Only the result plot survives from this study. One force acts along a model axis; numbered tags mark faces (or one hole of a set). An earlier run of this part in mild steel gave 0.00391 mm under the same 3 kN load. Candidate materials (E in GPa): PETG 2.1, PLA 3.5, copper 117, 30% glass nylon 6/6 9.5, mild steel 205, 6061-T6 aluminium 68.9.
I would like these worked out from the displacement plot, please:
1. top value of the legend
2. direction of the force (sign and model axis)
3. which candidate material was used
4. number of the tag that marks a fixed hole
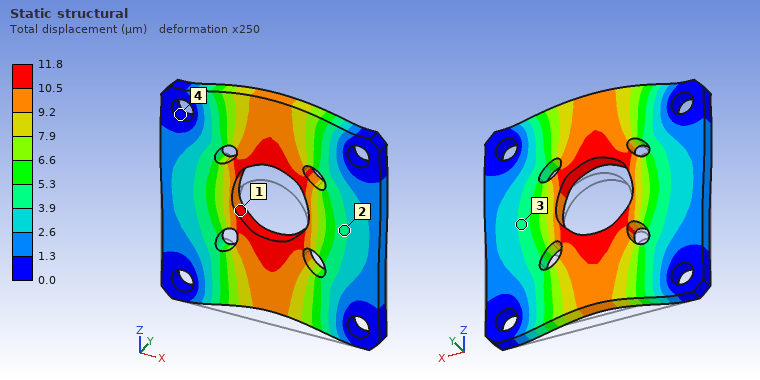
11.8 µm
+Z
6061-T6 aluminium
4
